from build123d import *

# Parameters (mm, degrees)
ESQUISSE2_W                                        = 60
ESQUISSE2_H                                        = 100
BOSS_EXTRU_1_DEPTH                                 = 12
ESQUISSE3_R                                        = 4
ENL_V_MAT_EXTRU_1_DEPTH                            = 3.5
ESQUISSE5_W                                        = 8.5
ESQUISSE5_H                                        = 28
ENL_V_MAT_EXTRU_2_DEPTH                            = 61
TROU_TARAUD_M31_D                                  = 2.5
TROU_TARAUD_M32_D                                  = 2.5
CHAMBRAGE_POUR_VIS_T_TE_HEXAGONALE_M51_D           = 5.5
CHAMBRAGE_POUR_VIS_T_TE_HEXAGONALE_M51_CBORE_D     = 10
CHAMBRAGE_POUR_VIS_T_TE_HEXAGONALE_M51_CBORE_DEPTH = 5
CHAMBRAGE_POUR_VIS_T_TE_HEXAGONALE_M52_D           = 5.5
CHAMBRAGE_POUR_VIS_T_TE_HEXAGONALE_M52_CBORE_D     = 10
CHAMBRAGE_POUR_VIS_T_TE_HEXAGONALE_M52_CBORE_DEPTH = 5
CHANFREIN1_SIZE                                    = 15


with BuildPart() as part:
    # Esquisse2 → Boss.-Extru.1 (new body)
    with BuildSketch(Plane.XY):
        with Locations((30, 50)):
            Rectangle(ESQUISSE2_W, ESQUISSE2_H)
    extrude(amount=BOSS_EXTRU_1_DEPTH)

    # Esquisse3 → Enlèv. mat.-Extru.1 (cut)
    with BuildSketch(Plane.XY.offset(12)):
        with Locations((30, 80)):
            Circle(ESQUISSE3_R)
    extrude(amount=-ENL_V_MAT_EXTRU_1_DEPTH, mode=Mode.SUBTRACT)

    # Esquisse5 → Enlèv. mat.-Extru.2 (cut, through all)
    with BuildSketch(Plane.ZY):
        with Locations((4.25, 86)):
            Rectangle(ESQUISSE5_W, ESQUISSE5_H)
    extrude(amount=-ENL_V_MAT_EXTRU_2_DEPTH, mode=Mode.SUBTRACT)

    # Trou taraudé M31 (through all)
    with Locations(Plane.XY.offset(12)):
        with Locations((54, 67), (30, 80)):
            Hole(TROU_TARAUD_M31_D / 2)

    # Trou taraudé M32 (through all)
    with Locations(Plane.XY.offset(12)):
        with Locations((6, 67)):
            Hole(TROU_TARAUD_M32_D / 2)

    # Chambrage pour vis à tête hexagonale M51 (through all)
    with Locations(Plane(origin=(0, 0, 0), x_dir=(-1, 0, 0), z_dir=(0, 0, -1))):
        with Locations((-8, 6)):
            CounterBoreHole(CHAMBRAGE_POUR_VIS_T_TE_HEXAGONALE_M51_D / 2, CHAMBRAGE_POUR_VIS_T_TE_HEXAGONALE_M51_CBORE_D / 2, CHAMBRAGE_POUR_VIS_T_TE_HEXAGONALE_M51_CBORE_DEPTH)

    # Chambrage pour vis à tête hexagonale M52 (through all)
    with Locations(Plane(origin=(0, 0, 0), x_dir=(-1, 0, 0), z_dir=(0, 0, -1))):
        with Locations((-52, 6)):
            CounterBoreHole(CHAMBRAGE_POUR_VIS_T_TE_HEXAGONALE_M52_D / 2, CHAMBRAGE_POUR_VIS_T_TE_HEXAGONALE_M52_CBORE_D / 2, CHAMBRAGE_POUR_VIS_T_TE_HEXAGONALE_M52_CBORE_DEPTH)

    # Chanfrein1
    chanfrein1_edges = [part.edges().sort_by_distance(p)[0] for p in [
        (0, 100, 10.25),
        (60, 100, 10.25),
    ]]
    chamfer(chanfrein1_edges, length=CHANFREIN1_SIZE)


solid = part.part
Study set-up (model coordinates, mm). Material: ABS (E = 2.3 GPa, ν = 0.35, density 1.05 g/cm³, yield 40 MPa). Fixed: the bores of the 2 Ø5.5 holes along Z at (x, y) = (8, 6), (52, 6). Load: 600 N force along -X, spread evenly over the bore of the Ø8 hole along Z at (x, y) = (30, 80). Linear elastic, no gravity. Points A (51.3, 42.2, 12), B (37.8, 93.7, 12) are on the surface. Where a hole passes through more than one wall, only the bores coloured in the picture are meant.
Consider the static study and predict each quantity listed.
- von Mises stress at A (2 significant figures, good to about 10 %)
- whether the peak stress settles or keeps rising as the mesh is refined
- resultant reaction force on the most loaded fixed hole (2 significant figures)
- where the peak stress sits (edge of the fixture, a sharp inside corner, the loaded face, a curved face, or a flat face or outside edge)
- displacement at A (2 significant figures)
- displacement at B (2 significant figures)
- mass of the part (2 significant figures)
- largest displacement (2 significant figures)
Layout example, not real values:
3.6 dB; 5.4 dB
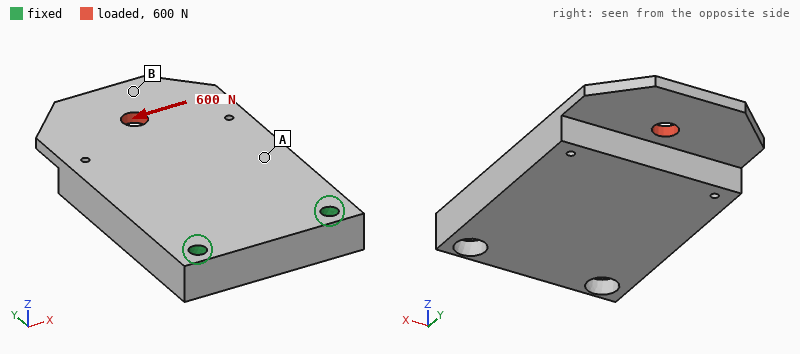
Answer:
3.8 MPa; keeps rising; 1.0 kN; edge of the fixture; 0.19 mm; 0.46 mm; 58 g; 0.50 mm
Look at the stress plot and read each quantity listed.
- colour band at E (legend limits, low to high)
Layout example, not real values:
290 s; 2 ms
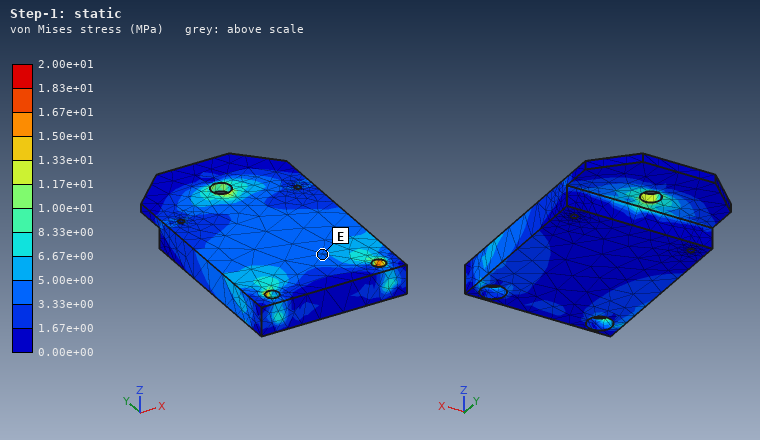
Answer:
3.33e+00 to 5.00e+00 MPa
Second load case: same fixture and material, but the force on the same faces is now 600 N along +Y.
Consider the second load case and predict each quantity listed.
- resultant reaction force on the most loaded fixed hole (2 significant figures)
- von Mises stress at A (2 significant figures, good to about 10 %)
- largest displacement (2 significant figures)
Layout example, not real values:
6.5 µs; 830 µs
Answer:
310 N; 2.6 MPa; 0.67 mm
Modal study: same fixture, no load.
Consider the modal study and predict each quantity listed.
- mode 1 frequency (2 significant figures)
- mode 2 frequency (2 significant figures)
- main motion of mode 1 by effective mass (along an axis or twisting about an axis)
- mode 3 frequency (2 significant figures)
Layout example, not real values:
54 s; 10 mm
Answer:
340 Hz; 1200 Hz; along Z; 1200 Hz
